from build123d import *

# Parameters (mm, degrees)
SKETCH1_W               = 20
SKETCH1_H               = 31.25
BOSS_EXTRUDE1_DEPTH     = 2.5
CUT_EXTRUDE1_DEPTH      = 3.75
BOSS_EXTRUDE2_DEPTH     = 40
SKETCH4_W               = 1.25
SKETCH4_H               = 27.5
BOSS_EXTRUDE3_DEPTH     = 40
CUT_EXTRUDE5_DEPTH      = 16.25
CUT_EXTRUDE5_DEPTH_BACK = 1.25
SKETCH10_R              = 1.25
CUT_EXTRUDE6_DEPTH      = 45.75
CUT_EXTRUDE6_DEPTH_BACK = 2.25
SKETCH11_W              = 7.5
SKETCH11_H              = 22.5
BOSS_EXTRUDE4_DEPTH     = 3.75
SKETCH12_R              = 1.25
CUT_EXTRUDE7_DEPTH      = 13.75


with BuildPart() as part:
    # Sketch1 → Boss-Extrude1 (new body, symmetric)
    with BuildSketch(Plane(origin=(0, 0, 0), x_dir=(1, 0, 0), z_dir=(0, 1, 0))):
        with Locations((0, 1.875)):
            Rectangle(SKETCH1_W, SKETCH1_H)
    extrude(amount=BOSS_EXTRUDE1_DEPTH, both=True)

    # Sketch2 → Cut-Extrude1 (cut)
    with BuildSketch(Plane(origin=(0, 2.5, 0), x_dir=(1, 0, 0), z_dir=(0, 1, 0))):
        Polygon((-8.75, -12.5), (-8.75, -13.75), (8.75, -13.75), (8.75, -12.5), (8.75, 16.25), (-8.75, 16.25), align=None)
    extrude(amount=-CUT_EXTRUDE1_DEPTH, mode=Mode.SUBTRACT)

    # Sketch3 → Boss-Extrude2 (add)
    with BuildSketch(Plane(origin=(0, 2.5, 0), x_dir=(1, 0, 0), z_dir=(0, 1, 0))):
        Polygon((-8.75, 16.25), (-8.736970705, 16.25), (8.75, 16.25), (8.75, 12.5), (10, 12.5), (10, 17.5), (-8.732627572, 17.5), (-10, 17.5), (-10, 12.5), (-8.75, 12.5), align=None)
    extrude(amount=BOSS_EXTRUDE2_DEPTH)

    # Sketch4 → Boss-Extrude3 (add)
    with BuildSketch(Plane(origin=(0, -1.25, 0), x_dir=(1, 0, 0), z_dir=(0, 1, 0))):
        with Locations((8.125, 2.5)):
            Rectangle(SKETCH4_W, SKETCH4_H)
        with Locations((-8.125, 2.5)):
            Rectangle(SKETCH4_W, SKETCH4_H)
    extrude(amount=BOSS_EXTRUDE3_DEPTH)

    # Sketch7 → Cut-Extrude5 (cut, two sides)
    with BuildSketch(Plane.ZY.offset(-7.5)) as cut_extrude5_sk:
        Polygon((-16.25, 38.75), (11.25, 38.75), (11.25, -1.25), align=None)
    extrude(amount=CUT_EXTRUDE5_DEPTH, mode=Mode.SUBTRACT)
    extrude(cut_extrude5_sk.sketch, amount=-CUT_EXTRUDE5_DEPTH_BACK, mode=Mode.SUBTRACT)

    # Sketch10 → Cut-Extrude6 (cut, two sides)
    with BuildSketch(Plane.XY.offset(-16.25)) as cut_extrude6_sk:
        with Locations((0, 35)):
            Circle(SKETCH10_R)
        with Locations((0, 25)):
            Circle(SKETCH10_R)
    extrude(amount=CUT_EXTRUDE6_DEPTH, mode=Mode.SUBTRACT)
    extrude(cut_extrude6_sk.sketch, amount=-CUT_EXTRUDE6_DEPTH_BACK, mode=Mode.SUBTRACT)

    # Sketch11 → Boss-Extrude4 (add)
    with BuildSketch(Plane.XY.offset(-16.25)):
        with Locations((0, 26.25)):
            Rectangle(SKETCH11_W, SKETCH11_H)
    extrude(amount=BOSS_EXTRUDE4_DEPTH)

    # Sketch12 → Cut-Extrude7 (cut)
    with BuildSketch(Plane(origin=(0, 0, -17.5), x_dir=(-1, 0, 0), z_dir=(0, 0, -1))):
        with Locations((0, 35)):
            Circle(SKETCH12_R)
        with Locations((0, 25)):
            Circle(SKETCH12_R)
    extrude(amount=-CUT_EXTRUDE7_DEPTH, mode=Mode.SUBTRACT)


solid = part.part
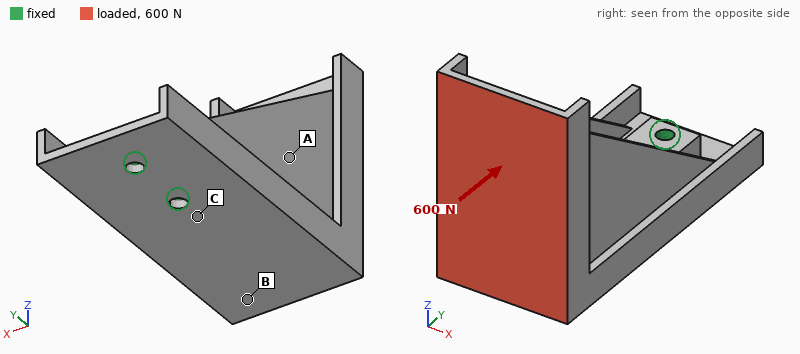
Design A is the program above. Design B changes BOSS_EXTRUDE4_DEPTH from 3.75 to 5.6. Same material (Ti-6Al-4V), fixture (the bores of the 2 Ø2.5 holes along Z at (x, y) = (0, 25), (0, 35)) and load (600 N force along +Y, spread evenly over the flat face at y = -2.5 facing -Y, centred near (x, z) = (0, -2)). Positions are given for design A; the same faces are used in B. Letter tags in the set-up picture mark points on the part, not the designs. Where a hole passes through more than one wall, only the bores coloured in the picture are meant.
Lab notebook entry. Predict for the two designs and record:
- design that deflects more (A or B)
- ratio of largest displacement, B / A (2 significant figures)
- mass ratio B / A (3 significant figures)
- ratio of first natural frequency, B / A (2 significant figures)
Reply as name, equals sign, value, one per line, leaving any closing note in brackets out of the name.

design that deflects more = A
ratio of largest displacement, B / A = 0.89
mass ratio B / A = 1.07
ratio of first natural frequency, B / A = 1.0
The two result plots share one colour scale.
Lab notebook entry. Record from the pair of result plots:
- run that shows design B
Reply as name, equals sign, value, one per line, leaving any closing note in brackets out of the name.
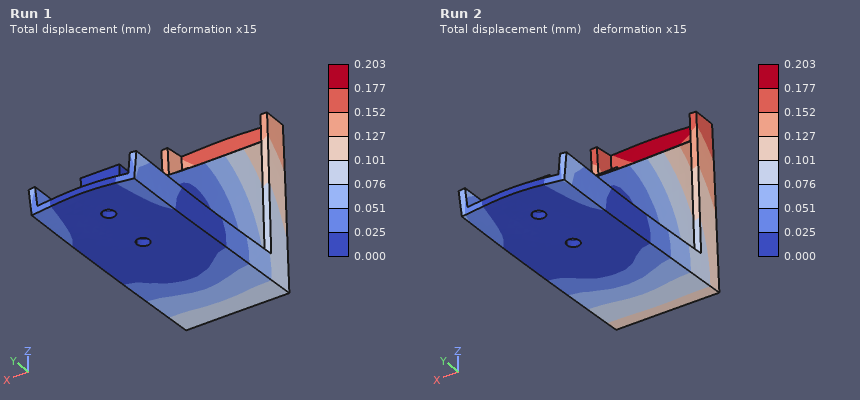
run that shows design B = Run 1
